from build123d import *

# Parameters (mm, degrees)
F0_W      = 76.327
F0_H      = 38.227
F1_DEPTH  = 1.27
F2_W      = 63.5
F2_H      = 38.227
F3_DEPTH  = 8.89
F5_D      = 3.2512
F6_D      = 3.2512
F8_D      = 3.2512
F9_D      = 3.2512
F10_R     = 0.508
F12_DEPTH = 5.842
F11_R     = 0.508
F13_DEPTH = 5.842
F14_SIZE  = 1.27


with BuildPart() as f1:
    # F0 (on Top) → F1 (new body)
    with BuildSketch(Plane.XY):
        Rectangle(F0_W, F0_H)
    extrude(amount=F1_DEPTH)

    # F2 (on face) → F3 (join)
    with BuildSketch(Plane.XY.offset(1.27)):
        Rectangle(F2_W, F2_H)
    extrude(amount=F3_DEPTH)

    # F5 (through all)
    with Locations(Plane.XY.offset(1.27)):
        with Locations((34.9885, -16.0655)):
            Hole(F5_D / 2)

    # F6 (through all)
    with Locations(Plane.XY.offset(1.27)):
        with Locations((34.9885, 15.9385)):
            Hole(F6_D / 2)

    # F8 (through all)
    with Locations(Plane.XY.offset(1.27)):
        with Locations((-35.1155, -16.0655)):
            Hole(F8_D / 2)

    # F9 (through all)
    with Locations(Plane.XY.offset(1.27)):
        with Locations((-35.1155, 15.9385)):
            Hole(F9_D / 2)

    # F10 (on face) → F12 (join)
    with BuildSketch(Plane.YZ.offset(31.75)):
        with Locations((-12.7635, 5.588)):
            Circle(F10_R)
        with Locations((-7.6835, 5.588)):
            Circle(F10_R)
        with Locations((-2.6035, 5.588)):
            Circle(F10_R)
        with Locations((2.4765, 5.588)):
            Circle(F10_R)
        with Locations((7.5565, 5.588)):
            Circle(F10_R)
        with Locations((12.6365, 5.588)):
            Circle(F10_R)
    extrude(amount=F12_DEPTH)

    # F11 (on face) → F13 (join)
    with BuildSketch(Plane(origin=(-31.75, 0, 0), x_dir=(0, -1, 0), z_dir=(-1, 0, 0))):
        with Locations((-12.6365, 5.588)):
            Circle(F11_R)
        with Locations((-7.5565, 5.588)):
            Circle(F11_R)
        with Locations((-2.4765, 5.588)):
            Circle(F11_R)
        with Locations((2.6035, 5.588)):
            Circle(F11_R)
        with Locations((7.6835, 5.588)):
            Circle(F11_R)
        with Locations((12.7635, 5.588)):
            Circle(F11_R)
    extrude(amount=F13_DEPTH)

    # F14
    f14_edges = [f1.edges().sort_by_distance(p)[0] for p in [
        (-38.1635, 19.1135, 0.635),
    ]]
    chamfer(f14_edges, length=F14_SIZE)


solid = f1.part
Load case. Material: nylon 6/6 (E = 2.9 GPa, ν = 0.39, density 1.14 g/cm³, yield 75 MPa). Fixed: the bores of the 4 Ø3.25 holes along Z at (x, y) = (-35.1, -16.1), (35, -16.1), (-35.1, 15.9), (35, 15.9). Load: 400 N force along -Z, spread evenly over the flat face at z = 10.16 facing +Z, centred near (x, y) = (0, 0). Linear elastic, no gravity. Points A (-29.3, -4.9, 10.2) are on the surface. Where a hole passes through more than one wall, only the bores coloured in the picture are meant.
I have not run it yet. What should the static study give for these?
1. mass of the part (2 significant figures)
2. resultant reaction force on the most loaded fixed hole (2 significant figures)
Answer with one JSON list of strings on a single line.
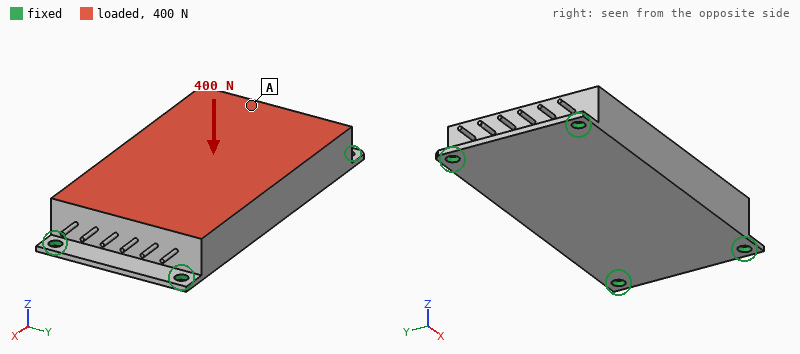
["29 g", "150 N"]
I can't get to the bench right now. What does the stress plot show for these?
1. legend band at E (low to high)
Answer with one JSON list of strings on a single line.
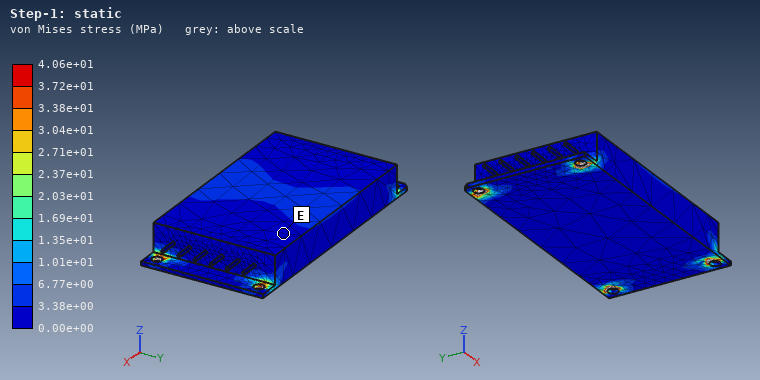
["0.00e+00 to 3.38e+00 MPa"]
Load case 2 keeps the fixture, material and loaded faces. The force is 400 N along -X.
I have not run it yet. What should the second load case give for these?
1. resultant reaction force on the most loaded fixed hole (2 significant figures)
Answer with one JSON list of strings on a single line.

["110 N"]
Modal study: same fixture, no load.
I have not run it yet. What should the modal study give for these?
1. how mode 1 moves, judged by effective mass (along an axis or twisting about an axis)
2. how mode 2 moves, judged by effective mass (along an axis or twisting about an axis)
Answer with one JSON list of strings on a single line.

["along Z", "along Y"]
